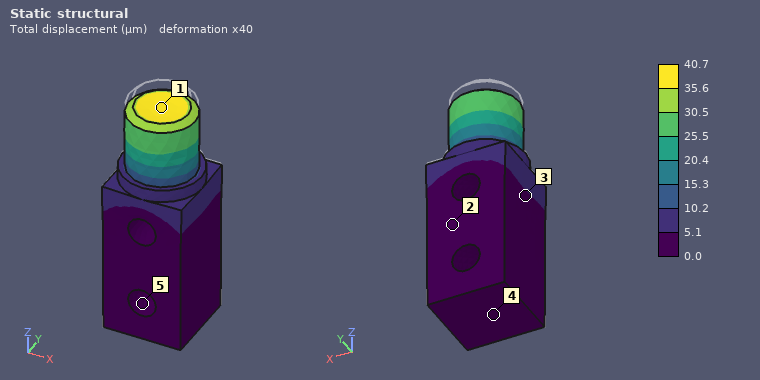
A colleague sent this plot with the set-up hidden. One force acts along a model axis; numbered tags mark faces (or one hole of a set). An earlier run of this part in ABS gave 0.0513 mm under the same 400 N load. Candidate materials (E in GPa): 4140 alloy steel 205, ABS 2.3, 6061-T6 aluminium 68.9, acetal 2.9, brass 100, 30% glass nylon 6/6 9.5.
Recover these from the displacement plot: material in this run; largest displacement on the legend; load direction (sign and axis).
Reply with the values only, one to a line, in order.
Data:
acetal
40.7 µm
-Z
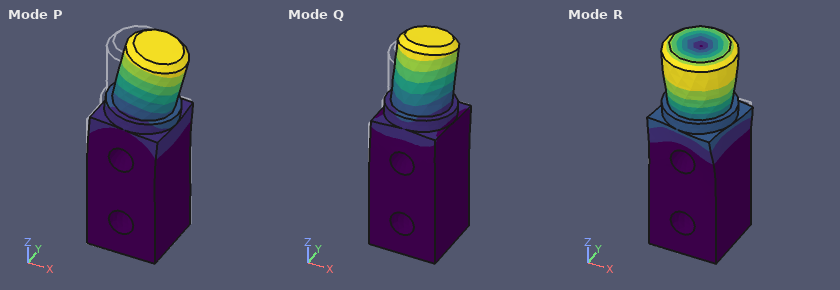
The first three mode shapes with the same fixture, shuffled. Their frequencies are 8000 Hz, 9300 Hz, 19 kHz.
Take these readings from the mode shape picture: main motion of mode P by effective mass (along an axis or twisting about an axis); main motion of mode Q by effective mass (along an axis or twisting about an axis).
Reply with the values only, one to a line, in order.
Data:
along X
along Y
